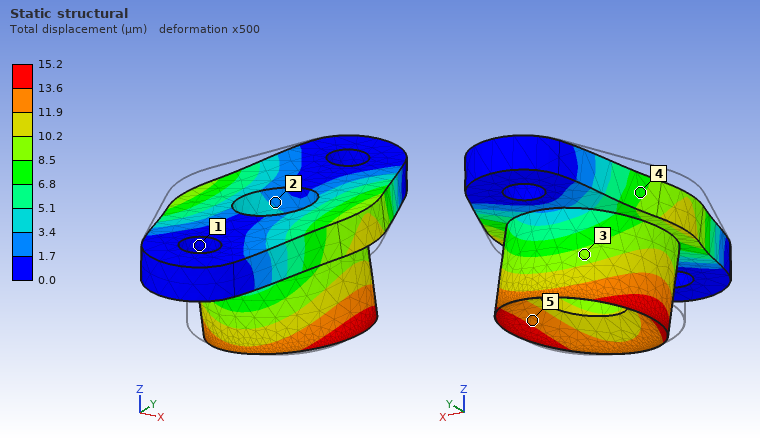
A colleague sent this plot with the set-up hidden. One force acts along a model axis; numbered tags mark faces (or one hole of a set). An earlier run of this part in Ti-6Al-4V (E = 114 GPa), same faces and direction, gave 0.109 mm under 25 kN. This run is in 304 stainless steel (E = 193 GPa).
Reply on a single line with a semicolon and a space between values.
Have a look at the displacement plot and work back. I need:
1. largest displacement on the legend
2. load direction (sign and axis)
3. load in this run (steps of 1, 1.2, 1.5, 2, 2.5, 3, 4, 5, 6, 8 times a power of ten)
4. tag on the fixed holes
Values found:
15.2 µm; +X; 6 kN; 1
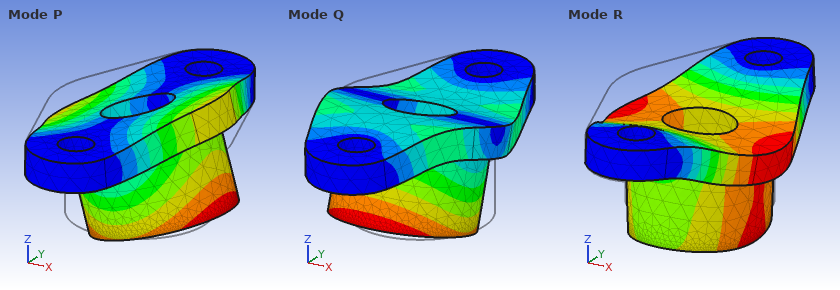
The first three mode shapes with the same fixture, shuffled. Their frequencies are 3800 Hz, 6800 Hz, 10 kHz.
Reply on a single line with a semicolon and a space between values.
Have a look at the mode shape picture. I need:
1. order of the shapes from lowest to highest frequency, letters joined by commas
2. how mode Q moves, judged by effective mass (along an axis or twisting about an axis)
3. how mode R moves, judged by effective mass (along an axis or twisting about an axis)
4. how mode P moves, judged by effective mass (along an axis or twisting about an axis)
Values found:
P, R, Q; along Y; along Z; along X
